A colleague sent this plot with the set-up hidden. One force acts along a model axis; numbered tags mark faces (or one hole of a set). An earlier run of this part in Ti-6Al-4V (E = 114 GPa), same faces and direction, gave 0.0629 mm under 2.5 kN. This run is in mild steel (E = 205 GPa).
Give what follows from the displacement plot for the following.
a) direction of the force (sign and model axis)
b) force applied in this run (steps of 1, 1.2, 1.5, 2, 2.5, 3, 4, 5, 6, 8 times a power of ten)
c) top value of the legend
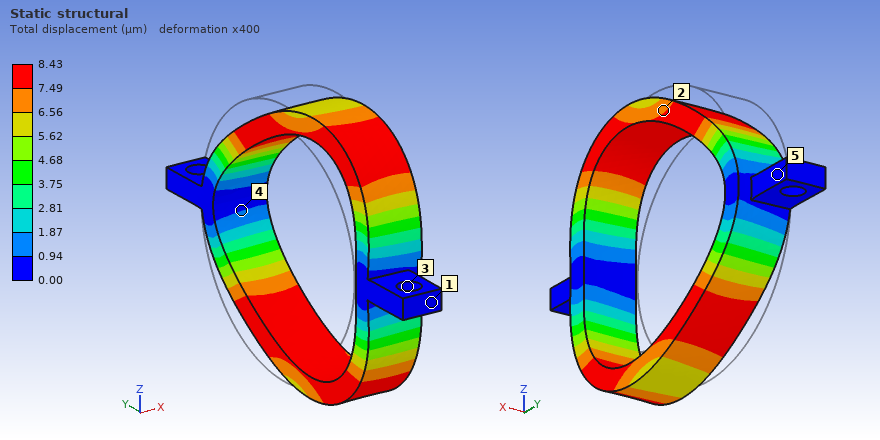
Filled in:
-Y
600 N
8.43 µm
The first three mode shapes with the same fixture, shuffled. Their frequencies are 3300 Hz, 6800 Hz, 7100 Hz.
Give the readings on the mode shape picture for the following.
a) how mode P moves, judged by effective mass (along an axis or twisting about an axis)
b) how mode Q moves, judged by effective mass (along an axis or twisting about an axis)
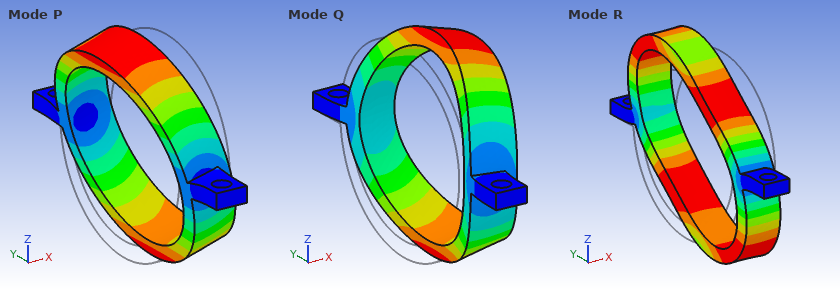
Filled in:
twisting about Y
along X
